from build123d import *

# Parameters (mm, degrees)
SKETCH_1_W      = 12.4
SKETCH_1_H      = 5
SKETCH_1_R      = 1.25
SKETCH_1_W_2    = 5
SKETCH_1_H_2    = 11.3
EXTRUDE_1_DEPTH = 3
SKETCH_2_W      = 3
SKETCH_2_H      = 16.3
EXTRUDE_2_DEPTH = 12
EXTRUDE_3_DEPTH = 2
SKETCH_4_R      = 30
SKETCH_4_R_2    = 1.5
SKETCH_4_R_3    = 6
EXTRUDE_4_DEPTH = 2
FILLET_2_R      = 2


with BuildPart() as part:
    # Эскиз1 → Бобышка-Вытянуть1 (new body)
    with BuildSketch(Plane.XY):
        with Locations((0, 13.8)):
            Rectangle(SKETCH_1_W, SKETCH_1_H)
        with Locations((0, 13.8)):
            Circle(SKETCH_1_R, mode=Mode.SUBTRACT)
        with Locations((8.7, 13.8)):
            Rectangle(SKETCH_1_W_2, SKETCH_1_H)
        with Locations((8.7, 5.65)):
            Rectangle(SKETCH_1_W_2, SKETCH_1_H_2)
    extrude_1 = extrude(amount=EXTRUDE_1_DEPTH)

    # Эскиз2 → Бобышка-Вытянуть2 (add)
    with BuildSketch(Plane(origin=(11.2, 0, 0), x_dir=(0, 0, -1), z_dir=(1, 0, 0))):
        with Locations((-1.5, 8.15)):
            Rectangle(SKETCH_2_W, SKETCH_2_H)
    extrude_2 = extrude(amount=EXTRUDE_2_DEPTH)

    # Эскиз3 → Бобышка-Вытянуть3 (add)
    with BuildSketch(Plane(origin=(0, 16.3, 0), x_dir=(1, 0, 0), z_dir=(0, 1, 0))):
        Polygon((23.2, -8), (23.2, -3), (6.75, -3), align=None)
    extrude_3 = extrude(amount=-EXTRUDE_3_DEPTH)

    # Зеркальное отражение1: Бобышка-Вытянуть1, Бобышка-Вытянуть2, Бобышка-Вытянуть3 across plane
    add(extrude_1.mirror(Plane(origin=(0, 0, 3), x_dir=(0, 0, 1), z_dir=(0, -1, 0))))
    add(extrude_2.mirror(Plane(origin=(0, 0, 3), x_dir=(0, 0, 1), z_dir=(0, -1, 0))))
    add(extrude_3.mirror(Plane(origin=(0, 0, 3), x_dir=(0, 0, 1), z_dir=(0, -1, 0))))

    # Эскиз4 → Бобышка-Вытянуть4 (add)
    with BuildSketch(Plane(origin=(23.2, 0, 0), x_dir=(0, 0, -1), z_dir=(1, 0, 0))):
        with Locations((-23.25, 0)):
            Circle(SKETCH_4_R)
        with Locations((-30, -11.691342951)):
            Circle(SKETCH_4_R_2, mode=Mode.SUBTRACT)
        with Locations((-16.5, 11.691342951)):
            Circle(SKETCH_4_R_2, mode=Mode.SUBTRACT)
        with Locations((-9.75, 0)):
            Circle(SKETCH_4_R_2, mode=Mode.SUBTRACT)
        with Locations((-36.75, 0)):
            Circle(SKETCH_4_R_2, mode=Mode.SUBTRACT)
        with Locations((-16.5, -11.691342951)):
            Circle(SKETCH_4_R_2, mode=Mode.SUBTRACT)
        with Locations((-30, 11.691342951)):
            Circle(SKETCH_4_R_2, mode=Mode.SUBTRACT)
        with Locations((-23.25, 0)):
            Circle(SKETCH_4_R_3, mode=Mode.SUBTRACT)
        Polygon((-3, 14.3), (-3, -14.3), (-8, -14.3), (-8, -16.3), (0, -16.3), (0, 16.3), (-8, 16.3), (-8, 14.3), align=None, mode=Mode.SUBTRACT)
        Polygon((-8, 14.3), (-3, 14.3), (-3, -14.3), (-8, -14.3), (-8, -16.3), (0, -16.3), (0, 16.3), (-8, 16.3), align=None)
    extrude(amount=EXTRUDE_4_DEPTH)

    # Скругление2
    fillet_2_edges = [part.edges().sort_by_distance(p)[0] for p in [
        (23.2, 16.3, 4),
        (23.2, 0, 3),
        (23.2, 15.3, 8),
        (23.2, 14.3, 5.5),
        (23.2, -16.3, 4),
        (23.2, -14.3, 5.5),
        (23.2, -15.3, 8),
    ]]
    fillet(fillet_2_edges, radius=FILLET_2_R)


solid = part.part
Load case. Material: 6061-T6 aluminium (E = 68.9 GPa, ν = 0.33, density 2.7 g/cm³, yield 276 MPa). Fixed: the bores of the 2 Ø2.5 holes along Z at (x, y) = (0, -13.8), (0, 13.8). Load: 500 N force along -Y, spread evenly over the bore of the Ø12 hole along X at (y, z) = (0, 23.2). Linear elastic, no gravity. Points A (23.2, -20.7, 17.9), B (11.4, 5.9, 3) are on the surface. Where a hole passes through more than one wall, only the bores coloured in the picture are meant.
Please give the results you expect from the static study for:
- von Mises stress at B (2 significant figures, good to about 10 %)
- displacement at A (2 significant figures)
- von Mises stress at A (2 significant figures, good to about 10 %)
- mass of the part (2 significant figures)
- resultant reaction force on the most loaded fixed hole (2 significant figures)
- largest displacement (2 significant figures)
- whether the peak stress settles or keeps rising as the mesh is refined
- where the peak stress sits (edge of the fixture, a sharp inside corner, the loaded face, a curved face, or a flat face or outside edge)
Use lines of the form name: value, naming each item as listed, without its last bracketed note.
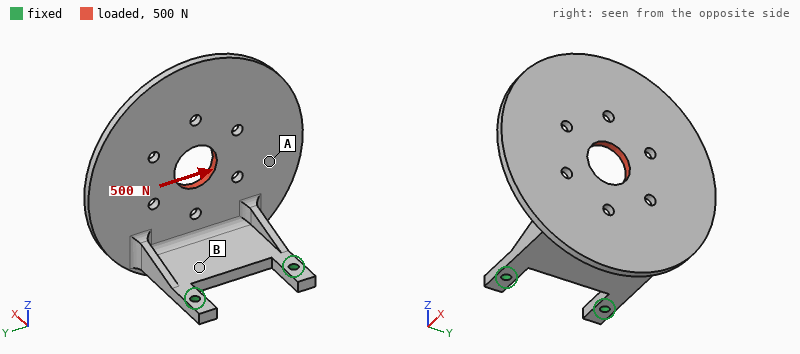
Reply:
von Mises stress at B: 140 MPa
displacement at A: 0.53 mm
von Mises stress at A: 39 MPa
mass of the part: 20 g
resultant reaction force on the most loaded fixed hole: 560 N
largest displacement: 1.00 mm
whether the peak stress settles or keeps rising as the mesh is refined: keeps rising
where the peak stress sits: edge of the fixture
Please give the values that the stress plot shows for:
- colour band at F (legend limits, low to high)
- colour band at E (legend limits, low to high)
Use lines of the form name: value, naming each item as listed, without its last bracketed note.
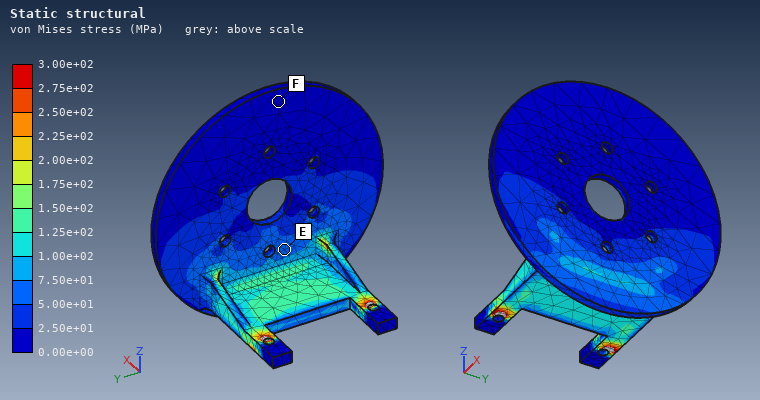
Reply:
colour band at F: 0.00e+00 to 2.50e+01 MPa
colour band at E: 5.00e+01 to 7.50e+01 MPa
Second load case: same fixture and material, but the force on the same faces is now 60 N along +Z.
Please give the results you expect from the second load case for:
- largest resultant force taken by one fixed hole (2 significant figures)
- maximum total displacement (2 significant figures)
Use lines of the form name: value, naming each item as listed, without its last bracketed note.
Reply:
largest resultant force taken by one fixed hole: 31 N
maximum total displacement: 0.38 mm
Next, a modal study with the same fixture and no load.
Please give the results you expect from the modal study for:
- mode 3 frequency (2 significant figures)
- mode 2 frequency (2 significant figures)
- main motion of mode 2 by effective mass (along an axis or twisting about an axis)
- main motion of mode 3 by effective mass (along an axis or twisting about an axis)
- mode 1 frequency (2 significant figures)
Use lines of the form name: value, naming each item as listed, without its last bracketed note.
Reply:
mode 3 frequency: 1400 Hz
mode 2 frequency: 990 Hz
main motion of mode 2 by effective mass: along Y
main motion of mode 3 by effective mass: along Z
mode 1 frequency: 450 Hz
